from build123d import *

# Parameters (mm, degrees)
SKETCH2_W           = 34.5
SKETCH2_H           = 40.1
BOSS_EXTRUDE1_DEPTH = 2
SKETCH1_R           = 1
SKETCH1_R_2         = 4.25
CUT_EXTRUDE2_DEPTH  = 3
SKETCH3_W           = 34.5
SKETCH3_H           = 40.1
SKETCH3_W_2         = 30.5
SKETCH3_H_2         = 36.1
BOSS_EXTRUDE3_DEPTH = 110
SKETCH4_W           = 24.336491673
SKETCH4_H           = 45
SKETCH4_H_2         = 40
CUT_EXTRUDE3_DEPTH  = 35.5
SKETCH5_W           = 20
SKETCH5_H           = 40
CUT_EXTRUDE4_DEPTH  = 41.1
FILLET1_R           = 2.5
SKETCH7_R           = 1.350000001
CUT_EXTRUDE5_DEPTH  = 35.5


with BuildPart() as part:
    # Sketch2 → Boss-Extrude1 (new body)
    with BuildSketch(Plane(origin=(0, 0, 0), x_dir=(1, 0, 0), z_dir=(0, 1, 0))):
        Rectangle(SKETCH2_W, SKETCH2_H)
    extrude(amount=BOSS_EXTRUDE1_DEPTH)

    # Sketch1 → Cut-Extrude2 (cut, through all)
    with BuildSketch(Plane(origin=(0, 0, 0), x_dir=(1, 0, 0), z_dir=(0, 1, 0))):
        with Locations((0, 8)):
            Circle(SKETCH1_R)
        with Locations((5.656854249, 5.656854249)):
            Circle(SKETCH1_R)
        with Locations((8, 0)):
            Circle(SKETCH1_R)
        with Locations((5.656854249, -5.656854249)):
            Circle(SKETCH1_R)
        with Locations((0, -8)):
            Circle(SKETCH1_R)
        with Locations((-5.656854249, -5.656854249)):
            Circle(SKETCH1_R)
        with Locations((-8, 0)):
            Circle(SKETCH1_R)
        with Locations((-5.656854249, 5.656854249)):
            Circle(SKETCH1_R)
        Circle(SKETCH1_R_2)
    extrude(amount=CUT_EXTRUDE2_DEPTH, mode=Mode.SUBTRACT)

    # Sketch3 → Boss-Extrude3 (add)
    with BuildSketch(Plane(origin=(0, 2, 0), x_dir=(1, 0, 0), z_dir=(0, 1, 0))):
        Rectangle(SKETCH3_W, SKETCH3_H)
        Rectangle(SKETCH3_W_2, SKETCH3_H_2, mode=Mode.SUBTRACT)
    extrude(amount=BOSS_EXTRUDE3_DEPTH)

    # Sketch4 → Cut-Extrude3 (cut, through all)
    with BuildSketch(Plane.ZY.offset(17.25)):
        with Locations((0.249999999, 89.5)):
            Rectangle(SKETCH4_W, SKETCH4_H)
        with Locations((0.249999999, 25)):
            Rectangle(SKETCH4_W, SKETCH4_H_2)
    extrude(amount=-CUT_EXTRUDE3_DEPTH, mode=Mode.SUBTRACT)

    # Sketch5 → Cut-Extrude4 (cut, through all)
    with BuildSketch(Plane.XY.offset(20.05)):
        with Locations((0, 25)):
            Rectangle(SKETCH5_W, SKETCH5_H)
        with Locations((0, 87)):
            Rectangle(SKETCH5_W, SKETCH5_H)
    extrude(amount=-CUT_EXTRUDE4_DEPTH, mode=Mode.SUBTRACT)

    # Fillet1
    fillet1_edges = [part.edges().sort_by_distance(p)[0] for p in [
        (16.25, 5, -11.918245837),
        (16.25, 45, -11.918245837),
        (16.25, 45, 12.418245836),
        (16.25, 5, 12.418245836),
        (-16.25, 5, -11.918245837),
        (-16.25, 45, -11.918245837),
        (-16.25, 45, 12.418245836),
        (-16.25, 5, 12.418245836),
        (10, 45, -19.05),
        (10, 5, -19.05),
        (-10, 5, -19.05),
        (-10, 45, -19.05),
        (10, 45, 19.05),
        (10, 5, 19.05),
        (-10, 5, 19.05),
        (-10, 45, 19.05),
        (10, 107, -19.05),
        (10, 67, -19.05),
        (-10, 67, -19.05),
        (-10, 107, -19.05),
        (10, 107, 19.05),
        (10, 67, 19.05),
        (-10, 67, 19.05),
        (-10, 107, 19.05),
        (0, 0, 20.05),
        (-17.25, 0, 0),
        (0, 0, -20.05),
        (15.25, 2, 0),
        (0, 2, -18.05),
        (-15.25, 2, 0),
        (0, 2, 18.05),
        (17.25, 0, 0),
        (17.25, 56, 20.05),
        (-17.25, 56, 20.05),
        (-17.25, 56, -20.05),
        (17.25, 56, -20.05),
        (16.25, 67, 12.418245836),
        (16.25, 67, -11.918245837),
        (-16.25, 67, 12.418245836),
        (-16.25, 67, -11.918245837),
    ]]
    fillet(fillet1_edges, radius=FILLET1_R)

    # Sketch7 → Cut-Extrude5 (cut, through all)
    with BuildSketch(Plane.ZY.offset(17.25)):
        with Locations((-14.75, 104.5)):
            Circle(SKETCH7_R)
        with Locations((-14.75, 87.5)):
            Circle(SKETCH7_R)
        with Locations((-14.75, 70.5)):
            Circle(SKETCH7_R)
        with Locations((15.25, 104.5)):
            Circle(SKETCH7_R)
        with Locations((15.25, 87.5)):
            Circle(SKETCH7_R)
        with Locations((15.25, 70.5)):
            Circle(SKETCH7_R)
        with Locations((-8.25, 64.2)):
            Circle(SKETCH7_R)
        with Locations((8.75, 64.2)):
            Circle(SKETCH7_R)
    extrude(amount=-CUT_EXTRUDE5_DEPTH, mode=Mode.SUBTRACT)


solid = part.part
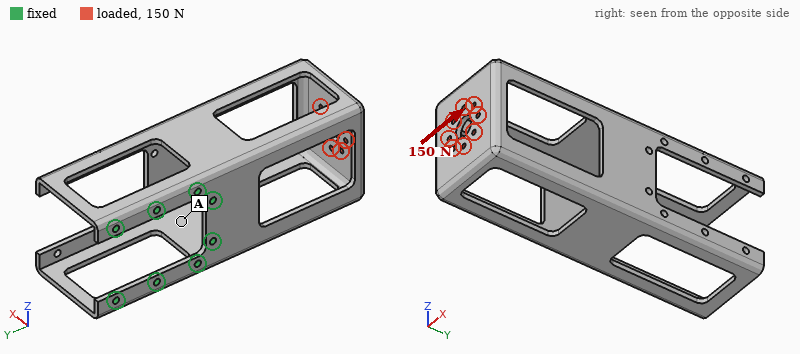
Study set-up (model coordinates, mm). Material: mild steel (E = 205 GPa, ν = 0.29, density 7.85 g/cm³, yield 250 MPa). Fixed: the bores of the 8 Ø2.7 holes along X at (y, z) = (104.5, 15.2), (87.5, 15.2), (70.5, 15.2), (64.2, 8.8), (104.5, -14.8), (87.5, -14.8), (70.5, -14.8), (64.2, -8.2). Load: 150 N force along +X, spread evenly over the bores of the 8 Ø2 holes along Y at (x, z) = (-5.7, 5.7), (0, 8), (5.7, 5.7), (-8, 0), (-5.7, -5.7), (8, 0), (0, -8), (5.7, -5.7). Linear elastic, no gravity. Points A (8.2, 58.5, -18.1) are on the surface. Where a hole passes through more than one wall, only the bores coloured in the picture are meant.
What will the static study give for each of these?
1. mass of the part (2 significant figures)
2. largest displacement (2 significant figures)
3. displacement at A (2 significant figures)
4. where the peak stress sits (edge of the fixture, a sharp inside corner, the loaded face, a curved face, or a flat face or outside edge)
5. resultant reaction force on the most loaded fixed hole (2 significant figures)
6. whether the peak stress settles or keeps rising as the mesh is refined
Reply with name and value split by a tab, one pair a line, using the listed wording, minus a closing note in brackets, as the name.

mass of the part	140 g
largest displacement	96 µm
displacement at A	26 µm
where the peak stress sits	edge of the fixture
resultant reaction force on the most loaded fixed hole	200 N
whether the peak stress settles or keeps rising as the mesh is refined	keeps rising
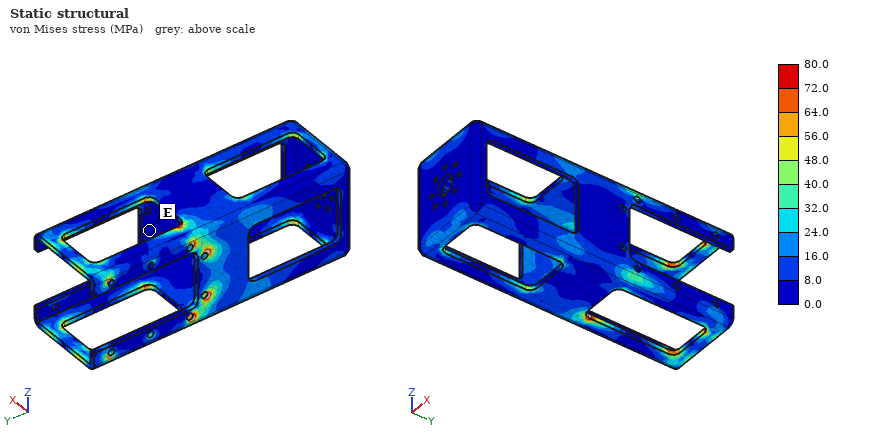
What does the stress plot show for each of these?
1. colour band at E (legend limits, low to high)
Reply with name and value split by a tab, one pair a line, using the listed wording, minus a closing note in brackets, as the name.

colour band at E	0.0 to 8.0 MPa
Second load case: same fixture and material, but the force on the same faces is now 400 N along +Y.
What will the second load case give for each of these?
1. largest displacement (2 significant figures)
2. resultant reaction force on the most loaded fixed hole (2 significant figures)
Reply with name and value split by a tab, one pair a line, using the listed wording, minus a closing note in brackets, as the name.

largest displacement	57 µm
resultant reaction force on the most loaded fixed hole	140 N
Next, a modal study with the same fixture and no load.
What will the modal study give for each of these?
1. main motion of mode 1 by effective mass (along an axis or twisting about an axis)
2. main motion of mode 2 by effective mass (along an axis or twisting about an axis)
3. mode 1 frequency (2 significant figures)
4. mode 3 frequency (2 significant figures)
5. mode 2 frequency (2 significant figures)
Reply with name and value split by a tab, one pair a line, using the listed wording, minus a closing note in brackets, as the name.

main motion of mode 1 by effective mass	along Z
main motion of mode 2 by effective mass	along X
mode 1 frequency	820 Hz
mode 3 frequency	1700 Hz
mode 2 frequency	930 Hz
